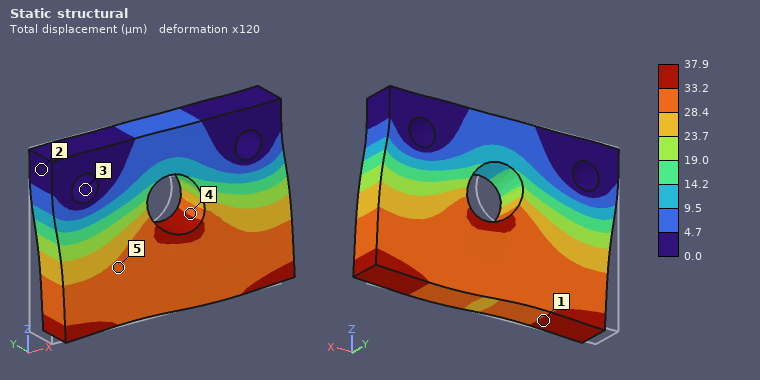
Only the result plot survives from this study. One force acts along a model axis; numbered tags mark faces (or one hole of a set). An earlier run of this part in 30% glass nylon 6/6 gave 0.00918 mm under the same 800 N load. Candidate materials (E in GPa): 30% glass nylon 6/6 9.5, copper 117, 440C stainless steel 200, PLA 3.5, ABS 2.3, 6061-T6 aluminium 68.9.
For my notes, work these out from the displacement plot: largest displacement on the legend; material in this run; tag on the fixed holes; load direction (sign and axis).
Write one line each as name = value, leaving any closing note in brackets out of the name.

largest displacement on the legend = 37.9 µm
material in this run = ABS
tag on the fixed holes = 3
load direction = +X
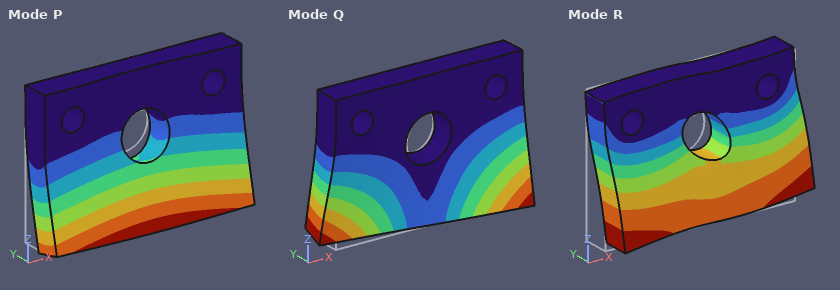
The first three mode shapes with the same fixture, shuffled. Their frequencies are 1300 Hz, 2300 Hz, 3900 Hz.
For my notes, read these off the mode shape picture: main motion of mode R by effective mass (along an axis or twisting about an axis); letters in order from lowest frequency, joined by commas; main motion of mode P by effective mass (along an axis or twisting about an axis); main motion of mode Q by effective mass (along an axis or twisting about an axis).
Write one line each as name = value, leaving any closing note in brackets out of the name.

main motion of mode R by effective mass = along X
letters in order from lowest frequency, joined by commas = P, Q, R
main motion of mode P by effective mass = along Y
main motion of mode Q by effective mass = twisting about Z
